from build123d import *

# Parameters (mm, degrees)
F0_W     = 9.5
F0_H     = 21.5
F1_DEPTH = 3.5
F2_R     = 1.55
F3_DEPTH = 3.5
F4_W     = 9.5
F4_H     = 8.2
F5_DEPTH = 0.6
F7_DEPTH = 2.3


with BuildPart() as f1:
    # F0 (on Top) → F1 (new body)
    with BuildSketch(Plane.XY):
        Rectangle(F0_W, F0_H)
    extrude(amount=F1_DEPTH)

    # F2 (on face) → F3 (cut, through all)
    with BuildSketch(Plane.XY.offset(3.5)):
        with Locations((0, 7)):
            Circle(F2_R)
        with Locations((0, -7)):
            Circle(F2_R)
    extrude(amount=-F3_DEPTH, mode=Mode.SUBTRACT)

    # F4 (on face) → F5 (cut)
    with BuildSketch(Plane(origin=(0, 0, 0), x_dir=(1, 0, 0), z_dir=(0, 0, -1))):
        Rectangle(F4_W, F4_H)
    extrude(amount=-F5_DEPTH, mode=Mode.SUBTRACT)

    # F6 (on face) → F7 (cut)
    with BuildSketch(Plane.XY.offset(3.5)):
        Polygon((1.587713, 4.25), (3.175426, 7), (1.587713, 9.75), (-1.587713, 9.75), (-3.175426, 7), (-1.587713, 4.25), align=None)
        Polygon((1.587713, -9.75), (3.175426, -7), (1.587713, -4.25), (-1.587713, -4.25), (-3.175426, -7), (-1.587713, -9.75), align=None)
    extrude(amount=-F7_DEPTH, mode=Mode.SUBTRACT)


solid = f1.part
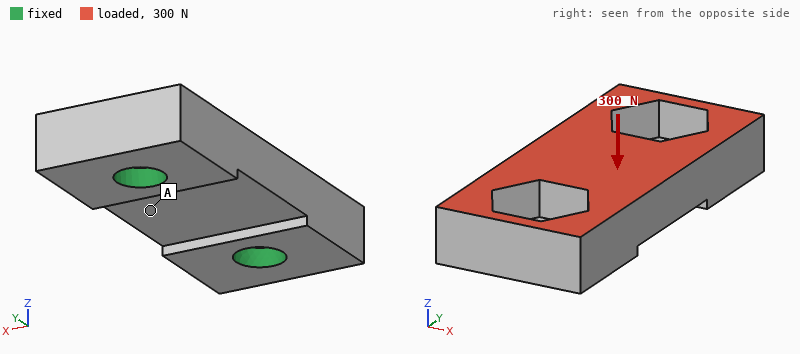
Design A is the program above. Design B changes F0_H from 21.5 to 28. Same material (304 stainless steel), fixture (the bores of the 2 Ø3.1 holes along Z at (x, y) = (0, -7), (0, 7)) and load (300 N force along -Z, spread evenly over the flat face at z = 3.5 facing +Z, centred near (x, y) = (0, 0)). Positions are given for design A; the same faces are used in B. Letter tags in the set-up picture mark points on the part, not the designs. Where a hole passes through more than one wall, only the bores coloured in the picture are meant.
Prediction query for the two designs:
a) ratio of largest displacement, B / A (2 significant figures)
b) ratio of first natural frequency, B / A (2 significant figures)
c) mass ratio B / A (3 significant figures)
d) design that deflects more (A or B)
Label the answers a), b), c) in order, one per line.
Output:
a) 1.4
b) 0.88
c) 1.41
d) B
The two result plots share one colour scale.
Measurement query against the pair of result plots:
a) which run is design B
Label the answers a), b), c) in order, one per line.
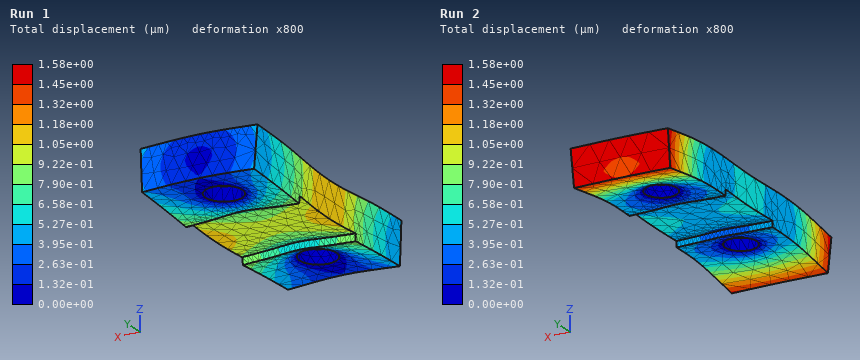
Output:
a) Run 2
